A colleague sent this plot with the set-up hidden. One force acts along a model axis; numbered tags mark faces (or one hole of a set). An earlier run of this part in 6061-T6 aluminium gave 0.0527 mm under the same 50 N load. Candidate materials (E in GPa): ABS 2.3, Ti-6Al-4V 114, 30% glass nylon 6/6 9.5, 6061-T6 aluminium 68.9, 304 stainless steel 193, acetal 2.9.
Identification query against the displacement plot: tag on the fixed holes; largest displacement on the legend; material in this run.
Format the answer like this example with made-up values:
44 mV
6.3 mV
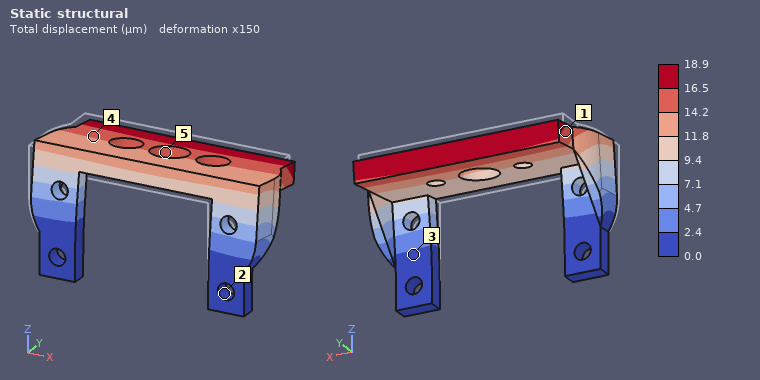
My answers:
2
18.9 µm
304 stainless steel
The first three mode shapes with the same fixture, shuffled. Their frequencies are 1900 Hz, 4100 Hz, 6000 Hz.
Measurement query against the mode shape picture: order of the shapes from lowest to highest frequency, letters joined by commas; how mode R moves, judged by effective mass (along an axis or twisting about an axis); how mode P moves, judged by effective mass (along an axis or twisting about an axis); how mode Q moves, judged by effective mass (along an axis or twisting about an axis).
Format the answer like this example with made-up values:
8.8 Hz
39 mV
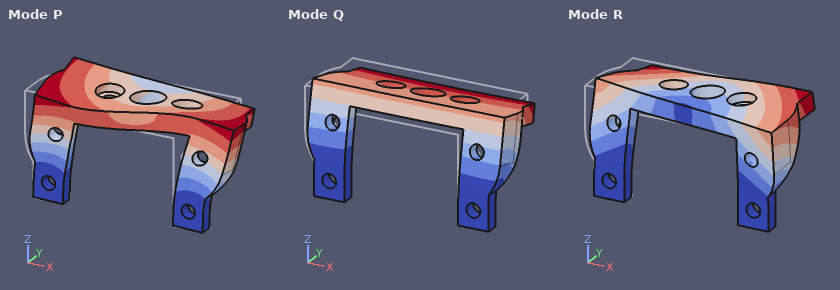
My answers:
Q, R, P
along X
along X
along Y
